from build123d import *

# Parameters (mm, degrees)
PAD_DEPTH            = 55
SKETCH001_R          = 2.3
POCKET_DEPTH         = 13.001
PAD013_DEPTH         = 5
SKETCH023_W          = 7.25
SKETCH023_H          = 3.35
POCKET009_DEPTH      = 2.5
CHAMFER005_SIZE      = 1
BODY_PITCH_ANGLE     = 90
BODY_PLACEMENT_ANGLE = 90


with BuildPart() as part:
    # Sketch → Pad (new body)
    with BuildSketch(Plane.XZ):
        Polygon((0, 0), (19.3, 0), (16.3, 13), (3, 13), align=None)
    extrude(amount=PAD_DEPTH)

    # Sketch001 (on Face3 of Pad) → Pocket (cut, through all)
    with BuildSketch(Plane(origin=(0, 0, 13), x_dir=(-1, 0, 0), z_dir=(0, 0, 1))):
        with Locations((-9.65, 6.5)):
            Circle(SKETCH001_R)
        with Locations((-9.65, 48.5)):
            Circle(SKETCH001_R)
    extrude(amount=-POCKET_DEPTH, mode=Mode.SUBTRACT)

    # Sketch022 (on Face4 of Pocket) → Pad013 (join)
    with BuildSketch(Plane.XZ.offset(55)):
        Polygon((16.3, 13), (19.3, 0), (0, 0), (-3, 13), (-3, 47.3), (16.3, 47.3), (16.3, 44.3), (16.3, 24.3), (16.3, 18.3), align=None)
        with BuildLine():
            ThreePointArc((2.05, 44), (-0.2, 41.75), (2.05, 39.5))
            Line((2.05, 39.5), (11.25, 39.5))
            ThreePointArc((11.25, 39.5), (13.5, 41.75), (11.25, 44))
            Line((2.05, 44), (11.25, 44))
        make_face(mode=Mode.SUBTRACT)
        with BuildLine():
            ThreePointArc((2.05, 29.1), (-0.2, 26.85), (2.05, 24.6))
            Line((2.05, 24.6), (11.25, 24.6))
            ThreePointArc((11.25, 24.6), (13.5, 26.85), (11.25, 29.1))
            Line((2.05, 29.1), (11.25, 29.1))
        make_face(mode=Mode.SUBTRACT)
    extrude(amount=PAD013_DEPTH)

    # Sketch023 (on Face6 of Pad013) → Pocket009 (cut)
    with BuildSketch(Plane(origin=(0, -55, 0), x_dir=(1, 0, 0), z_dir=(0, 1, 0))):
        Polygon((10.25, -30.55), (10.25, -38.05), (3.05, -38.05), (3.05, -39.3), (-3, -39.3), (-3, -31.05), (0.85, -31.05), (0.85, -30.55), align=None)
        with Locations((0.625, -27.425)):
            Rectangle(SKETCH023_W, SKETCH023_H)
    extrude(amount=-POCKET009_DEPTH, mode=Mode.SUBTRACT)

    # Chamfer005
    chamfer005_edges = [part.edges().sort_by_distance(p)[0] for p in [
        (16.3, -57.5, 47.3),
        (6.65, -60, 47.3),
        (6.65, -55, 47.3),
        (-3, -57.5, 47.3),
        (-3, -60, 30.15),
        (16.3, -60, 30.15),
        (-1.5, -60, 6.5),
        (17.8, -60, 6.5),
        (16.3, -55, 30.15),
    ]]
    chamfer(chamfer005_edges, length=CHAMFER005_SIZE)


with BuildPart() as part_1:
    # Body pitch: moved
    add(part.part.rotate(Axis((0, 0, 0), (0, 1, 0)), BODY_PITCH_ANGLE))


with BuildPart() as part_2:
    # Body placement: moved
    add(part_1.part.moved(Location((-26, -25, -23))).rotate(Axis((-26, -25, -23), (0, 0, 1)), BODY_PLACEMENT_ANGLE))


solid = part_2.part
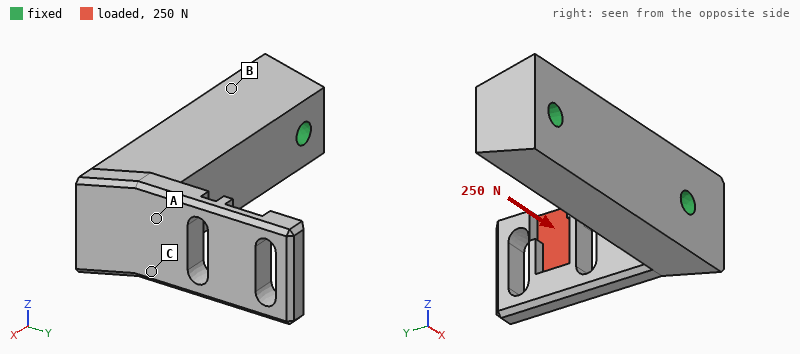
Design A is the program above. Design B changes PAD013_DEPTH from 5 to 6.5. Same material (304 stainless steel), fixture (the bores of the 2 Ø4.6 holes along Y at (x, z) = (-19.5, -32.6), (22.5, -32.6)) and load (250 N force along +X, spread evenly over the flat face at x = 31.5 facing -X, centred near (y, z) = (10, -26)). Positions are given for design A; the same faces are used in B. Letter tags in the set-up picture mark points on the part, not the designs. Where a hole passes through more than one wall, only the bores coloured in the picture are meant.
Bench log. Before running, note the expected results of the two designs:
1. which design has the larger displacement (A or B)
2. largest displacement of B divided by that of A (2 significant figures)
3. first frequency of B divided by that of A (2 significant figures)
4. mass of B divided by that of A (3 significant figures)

A
0.46
1.3
1.08
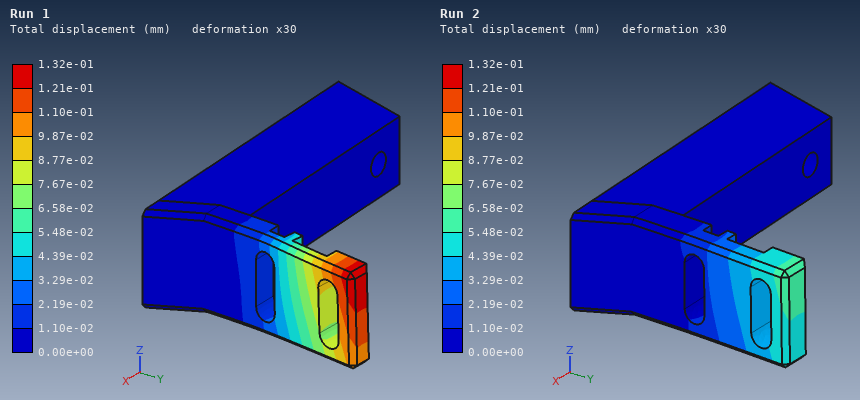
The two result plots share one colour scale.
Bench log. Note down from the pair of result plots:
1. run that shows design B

Run 2
